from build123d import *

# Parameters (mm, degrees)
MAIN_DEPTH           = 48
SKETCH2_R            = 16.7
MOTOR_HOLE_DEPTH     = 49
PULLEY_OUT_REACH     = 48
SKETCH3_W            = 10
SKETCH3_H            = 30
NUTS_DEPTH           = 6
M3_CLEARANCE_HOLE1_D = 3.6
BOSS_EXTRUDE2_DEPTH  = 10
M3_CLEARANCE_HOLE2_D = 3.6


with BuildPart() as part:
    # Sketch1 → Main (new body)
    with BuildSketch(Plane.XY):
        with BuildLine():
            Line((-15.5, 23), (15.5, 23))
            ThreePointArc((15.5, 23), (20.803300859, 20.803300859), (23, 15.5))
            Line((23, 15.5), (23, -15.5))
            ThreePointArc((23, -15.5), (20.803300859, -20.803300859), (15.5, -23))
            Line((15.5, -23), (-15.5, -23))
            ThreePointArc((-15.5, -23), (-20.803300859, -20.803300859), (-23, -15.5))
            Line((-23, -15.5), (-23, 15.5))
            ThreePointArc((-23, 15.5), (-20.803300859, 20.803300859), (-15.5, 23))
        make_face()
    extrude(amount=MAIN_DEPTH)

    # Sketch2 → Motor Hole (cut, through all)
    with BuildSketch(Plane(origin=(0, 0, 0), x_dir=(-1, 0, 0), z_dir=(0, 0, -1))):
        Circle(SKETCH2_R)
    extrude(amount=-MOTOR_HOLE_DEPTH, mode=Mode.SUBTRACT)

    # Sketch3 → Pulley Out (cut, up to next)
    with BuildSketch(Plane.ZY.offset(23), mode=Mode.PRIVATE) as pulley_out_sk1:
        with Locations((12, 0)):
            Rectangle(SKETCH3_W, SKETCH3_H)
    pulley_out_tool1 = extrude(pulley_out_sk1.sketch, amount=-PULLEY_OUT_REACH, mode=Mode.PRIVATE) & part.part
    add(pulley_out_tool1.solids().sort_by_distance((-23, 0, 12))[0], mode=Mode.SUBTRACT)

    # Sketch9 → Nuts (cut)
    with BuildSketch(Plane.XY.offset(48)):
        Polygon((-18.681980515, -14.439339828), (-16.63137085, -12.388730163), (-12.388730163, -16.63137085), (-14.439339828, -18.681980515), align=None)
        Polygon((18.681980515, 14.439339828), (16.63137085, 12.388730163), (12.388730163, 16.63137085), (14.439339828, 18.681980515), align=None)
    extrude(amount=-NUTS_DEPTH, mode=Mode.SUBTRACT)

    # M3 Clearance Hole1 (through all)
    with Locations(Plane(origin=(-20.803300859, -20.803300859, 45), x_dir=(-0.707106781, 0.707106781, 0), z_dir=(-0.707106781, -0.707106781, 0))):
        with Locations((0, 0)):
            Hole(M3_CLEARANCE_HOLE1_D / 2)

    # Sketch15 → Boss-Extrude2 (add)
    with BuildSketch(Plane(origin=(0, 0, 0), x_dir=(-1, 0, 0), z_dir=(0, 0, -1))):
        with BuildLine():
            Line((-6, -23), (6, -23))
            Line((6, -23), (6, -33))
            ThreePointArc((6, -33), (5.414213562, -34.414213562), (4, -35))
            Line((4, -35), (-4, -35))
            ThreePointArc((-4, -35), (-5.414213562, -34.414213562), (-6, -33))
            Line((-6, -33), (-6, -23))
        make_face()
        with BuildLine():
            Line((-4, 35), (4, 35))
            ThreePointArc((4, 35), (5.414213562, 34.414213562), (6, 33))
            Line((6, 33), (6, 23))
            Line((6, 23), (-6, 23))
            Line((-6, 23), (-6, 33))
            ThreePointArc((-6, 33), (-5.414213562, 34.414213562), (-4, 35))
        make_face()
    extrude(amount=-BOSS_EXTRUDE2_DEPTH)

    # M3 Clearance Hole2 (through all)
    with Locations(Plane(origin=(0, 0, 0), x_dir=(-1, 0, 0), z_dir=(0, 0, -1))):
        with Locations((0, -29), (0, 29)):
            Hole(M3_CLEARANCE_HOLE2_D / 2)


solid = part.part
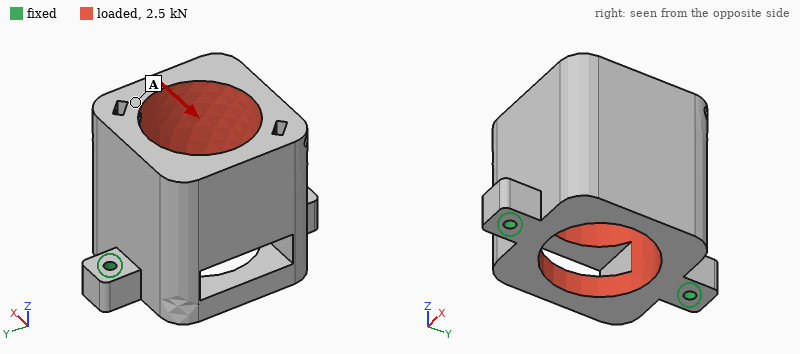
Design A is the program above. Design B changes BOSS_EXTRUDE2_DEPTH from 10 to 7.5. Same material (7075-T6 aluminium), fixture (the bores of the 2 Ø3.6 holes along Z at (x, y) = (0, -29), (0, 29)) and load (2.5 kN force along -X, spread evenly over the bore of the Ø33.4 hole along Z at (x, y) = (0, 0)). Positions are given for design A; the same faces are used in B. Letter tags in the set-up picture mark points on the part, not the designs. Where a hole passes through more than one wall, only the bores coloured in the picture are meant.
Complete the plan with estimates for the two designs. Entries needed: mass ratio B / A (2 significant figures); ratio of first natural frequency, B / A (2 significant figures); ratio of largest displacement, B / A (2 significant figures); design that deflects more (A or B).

0.99
0.73
1.9
B
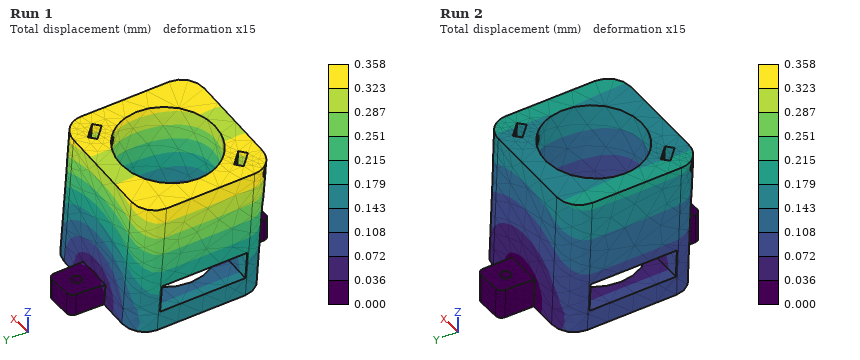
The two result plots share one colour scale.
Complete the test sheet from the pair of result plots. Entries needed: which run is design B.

Run 1
